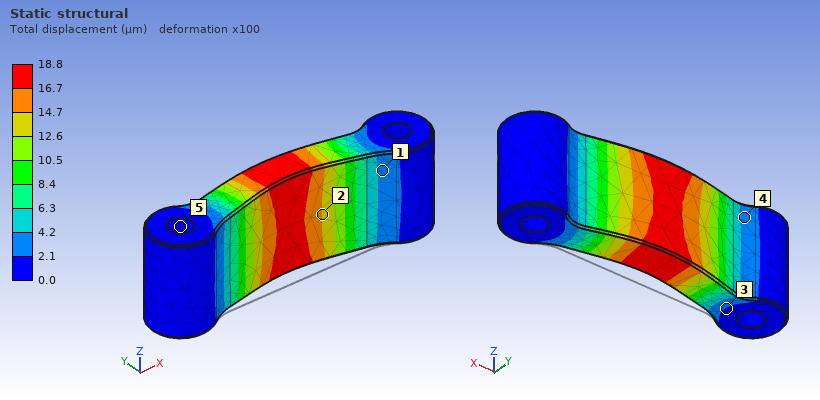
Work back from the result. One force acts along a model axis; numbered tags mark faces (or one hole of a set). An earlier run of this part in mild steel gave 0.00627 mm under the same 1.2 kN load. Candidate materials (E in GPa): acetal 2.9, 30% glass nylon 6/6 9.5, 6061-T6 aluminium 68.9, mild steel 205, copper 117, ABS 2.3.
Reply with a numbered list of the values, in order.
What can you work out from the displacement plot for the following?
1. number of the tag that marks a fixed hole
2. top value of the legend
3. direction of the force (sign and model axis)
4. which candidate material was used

1. 5
2. 18.8 µm
3. +Y
4. 6061-T6 aluminium
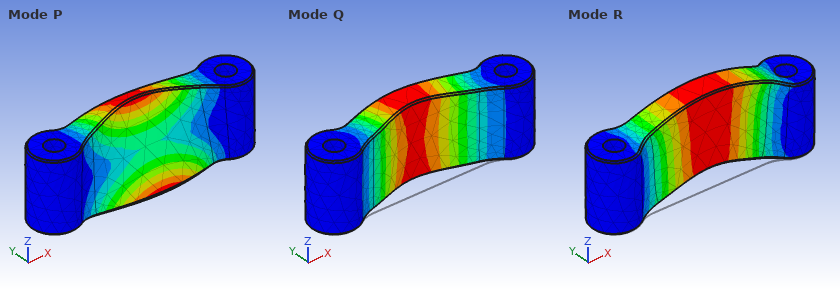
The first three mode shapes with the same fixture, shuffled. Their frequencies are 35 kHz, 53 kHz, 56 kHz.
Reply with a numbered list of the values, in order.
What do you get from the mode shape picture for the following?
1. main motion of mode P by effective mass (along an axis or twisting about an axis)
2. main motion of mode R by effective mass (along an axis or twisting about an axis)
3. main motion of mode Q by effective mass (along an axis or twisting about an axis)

1. twisting about X
2. along Z
3. along Y
